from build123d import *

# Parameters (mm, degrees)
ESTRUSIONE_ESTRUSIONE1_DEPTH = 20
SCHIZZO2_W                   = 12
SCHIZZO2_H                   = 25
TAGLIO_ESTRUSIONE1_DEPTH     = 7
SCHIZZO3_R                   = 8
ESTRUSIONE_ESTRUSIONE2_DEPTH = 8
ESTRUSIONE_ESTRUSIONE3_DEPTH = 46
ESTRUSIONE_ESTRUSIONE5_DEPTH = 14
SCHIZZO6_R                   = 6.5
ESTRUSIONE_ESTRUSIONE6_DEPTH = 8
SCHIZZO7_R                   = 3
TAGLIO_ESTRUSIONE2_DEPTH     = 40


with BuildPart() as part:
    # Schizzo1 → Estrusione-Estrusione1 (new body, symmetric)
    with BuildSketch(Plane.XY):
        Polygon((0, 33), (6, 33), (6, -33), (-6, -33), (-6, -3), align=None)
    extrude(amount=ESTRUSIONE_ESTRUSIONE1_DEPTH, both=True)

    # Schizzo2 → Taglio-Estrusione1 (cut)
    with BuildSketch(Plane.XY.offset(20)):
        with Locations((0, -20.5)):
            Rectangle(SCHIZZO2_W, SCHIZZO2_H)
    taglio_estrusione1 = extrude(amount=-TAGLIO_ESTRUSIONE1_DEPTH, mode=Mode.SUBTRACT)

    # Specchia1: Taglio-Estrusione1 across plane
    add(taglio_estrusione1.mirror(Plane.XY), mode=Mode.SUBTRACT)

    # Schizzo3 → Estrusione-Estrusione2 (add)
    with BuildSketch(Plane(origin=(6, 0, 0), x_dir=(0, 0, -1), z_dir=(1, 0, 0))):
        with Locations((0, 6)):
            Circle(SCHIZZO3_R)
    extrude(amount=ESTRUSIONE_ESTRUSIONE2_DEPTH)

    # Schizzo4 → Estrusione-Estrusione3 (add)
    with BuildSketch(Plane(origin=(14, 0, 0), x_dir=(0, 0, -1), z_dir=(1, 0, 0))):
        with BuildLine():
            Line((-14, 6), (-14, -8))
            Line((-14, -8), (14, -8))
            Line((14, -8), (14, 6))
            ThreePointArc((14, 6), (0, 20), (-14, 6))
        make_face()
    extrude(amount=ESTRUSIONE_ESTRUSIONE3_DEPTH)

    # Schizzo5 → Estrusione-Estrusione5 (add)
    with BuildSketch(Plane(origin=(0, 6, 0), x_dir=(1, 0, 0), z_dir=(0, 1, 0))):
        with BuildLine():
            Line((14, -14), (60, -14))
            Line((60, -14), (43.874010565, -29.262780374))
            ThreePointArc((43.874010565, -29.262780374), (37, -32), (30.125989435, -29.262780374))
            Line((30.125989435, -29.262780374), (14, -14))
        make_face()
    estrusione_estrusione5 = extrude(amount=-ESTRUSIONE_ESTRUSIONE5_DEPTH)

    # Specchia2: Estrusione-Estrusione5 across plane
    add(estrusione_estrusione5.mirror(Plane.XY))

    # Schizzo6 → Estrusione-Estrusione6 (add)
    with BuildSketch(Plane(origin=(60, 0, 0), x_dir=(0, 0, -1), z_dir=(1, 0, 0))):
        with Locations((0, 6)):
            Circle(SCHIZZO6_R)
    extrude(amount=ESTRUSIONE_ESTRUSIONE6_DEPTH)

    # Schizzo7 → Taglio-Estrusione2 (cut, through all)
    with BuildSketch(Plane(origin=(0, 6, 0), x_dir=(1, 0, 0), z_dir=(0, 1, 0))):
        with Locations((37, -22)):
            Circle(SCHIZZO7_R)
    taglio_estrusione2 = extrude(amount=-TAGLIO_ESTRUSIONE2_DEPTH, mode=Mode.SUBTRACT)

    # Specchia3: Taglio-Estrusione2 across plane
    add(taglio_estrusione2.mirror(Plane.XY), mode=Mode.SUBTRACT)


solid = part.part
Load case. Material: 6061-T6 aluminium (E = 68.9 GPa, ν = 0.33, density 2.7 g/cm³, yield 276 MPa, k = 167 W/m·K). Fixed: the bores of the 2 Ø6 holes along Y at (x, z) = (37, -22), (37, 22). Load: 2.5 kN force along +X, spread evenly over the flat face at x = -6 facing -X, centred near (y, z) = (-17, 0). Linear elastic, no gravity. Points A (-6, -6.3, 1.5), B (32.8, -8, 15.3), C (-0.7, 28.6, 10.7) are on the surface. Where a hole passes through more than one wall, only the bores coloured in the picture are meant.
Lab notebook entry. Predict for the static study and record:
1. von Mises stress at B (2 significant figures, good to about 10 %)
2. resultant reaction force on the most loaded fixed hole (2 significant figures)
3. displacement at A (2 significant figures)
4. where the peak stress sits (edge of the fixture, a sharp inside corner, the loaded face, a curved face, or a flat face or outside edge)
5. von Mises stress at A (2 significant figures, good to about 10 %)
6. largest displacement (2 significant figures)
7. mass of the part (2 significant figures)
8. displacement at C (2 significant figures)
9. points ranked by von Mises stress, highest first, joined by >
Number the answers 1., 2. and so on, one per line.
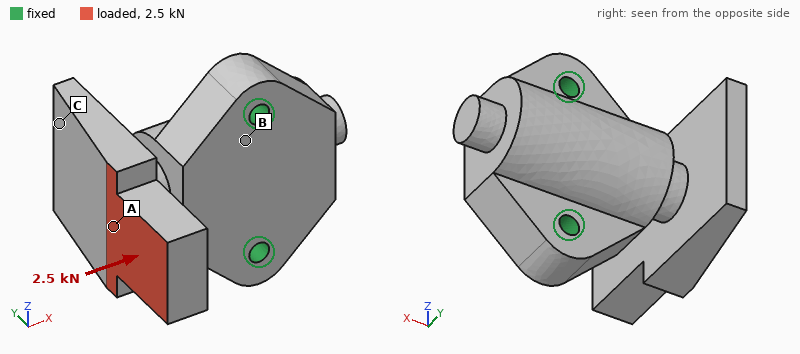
1. 22 MPa
2. 1.4 kN
3. 0.11 mm
4. a curved face
5. 38 MPa
6. 0.26 mm
7. 190 g
8. 0.12 mm
9. A > B > C
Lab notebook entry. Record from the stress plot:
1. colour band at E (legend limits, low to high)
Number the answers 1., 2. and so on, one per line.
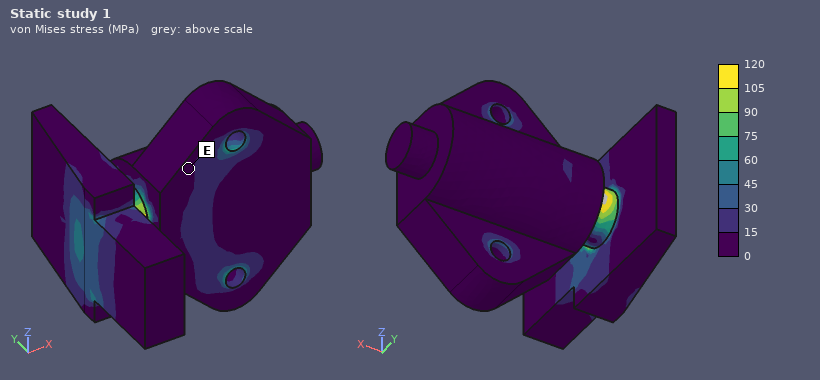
1. 0 to 15 MPa
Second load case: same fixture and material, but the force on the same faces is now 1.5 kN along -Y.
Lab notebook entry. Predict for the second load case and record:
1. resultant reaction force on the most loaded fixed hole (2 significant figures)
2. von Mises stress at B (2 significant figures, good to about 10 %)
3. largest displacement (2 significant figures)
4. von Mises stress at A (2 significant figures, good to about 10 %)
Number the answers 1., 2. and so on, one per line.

1. 900 N
2. 25 MPa
3. 0.14 mm
4. 15 MPa
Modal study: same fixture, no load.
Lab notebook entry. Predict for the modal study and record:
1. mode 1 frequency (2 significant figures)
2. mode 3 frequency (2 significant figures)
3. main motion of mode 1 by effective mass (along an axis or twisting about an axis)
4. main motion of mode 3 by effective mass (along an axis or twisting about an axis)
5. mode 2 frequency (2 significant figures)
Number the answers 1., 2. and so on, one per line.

1. 2700 Hz
2. 4900 Hz
3. along Y
4. along Z
5. 3100 Hz
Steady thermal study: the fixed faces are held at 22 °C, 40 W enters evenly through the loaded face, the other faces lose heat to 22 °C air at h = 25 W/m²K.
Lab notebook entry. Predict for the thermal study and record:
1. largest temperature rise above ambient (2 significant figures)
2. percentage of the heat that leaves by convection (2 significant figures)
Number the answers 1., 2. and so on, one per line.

1. 37 K
2. 11 %
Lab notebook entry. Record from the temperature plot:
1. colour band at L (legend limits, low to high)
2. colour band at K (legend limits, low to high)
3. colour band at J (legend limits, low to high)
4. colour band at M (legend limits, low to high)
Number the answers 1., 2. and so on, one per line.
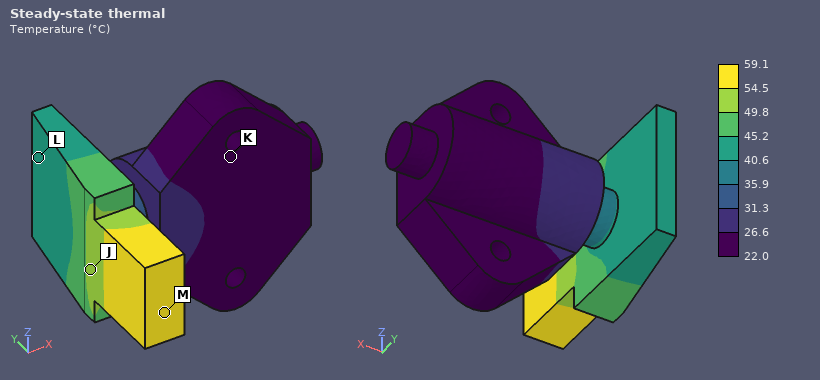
1. 40.6 to 45.2 °C
2. 22.0 to 26.6 °C
3. 49.8 to 54.5 °C
4. 54.5 to 59.1 °C
